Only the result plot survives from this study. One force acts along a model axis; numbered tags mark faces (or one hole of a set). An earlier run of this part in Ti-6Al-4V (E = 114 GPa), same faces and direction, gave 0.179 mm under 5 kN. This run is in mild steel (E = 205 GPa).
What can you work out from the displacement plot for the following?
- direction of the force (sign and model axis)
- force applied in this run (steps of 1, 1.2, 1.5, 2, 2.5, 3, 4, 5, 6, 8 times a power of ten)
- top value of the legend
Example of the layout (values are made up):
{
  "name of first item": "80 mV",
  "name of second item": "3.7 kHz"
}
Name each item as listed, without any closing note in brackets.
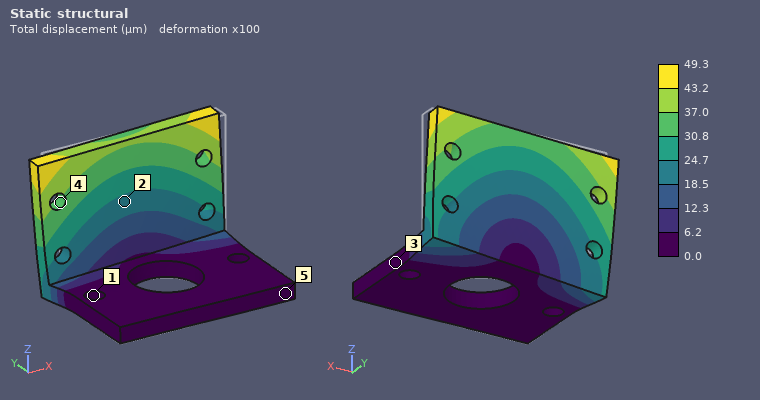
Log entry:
{
  "direction of the force": "-X",
  "force applied in this run": "2.5 kN",
  "top value of the legend": "49.3 µm"
}
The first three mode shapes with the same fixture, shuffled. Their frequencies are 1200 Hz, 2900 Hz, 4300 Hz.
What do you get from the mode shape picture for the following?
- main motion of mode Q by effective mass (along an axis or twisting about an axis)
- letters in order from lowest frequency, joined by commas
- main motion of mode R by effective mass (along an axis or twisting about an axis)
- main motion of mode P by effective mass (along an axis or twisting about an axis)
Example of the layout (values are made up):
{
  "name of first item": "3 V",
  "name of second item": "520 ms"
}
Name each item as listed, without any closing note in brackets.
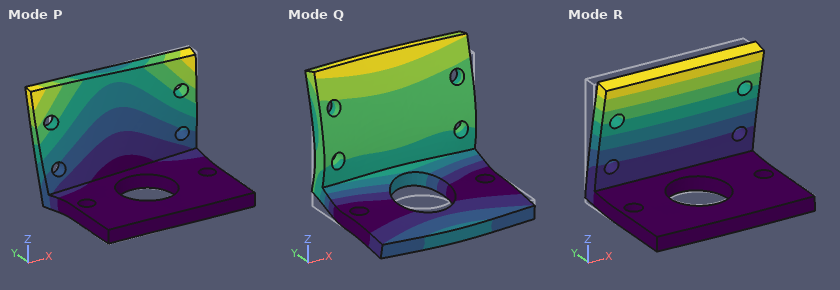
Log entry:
{
  "main motion of mode Q by effective mass": "along Z",
  "letters in order from lowest frequency, joined by commas": "R, P, Q",
  "main motion of mode R by effective mass": "along Y",
  "main motion of mode P by effective mass": "along X"
}
